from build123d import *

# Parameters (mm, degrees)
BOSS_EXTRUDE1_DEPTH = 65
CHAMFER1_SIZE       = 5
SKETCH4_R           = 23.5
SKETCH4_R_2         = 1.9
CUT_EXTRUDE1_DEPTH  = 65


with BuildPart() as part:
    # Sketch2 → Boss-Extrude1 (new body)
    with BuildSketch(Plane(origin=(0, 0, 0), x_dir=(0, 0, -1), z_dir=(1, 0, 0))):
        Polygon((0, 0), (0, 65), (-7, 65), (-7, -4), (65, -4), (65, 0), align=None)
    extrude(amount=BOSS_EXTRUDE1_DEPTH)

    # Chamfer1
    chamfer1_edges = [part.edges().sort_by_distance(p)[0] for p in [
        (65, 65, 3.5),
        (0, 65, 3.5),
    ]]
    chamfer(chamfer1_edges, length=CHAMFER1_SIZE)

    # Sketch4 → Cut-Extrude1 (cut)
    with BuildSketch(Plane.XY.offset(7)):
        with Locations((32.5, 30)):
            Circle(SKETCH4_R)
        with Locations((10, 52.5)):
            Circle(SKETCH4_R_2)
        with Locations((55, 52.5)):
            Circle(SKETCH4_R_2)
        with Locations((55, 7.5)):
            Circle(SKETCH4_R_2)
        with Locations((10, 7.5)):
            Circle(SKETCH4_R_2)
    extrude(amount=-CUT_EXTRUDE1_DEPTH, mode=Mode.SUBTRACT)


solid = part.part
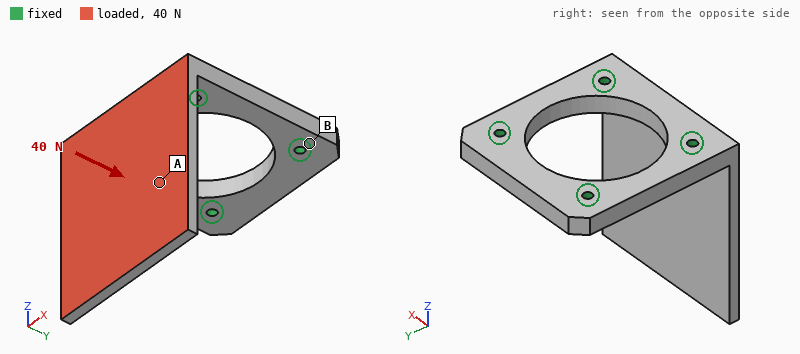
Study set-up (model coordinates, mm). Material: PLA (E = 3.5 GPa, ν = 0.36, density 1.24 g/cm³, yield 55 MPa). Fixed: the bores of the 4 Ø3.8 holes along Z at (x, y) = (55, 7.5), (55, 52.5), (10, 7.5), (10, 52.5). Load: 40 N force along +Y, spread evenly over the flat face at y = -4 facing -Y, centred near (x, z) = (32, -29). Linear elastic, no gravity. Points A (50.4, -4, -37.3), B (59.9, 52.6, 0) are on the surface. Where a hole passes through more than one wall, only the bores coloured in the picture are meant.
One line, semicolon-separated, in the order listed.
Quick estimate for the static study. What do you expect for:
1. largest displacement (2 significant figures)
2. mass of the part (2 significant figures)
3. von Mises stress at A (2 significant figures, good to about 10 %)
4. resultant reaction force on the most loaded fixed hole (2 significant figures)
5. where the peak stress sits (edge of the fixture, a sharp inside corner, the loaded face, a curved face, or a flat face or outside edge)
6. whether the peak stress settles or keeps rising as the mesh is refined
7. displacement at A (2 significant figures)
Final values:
1.3 mm; 44 g; 1.2 MPa; 26 N; edge of the fixture; keeps rising; 0.61 mm
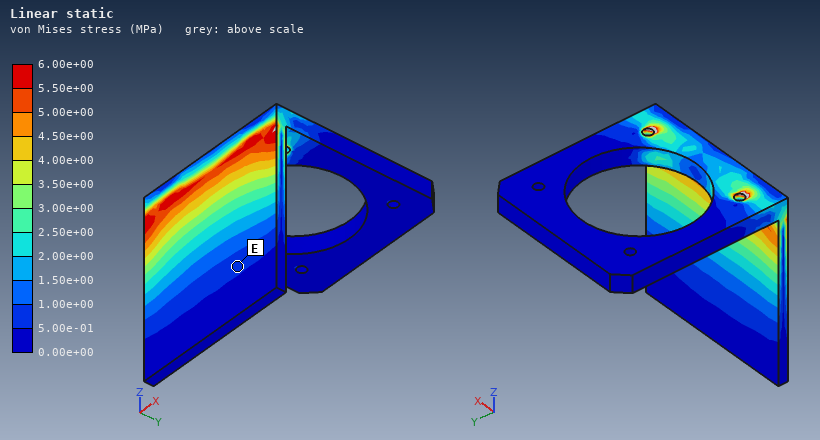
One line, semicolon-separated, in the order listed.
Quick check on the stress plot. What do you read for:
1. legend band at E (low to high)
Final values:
5.00e-01 to 1.00e+00 MPa
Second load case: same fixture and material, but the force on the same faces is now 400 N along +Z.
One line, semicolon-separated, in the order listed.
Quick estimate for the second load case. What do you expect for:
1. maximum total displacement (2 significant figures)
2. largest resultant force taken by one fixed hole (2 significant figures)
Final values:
1.4 mm; 210 N
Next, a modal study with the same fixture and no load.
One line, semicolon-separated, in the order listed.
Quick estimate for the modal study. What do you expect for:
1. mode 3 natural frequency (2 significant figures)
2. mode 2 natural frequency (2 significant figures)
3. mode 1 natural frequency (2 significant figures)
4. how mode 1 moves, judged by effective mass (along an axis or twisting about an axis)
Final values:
1400 Hz; 590 Hz; 230 Hz; along Y
